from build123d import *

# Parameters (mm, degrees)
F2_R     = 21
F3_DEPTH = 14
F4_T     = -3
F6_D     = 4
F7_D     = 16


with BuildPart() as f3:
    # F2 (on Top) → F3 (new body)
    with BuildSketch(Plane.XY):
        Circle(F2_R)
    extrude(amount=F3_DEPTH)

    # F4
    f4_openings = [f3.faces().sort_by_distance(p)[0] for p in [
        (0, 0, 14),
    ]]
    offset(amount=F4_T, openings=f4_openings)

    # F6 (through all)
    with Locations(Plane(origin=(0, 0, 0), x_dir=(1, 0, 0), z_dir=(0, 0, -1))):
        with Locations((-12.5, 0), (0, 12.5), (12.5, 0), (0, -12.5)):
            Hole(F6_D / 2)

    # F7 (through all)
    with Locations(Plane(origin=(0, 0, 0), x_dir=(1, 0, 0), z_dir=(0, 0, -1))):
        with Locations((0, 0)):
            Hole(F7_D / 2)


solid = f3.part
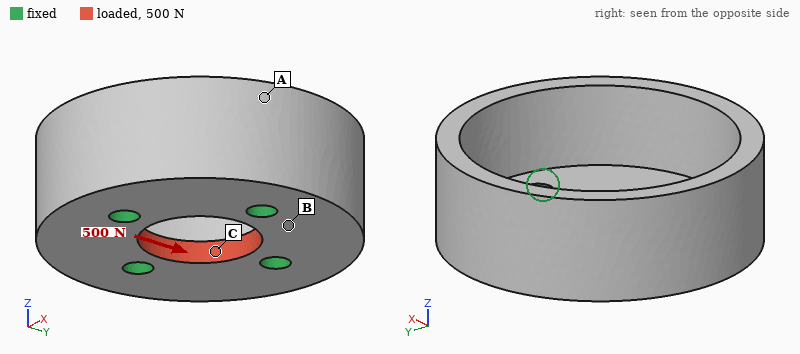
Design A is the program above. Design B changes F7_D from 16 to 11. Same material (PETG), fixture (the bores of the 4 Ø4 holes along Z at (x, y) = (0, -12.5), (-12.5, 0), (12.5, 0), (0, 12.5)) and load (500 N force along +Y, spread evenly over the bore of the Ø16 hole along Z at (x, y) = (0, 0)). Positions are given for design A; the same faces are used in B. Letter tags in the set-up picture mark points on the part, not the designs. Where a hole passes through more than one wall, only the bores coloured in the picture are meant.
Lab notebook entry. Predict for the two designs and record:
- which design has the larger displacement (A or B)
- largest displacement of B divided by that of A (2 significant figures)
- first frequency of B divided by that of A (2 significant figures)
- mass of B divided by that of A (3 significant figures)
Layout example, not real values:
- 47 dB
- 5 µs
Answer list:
- B
- 1.4
- 1.0
- 1.04
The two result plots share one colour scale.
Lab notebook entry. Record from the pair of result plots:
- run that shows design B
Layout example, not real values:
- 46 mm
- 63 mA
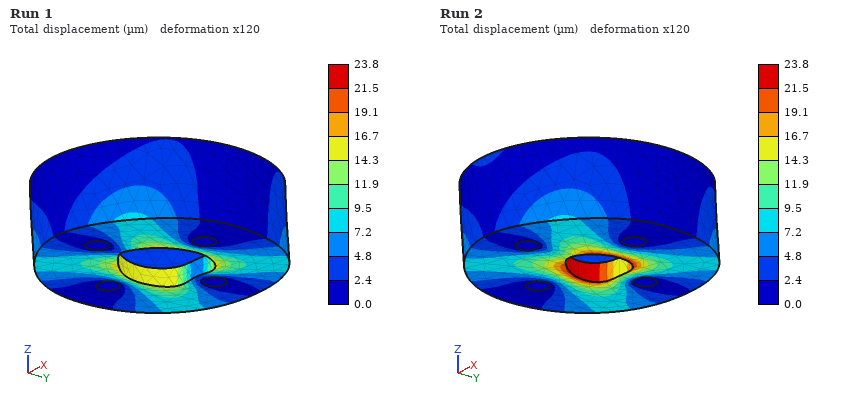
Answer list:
- Run 2
